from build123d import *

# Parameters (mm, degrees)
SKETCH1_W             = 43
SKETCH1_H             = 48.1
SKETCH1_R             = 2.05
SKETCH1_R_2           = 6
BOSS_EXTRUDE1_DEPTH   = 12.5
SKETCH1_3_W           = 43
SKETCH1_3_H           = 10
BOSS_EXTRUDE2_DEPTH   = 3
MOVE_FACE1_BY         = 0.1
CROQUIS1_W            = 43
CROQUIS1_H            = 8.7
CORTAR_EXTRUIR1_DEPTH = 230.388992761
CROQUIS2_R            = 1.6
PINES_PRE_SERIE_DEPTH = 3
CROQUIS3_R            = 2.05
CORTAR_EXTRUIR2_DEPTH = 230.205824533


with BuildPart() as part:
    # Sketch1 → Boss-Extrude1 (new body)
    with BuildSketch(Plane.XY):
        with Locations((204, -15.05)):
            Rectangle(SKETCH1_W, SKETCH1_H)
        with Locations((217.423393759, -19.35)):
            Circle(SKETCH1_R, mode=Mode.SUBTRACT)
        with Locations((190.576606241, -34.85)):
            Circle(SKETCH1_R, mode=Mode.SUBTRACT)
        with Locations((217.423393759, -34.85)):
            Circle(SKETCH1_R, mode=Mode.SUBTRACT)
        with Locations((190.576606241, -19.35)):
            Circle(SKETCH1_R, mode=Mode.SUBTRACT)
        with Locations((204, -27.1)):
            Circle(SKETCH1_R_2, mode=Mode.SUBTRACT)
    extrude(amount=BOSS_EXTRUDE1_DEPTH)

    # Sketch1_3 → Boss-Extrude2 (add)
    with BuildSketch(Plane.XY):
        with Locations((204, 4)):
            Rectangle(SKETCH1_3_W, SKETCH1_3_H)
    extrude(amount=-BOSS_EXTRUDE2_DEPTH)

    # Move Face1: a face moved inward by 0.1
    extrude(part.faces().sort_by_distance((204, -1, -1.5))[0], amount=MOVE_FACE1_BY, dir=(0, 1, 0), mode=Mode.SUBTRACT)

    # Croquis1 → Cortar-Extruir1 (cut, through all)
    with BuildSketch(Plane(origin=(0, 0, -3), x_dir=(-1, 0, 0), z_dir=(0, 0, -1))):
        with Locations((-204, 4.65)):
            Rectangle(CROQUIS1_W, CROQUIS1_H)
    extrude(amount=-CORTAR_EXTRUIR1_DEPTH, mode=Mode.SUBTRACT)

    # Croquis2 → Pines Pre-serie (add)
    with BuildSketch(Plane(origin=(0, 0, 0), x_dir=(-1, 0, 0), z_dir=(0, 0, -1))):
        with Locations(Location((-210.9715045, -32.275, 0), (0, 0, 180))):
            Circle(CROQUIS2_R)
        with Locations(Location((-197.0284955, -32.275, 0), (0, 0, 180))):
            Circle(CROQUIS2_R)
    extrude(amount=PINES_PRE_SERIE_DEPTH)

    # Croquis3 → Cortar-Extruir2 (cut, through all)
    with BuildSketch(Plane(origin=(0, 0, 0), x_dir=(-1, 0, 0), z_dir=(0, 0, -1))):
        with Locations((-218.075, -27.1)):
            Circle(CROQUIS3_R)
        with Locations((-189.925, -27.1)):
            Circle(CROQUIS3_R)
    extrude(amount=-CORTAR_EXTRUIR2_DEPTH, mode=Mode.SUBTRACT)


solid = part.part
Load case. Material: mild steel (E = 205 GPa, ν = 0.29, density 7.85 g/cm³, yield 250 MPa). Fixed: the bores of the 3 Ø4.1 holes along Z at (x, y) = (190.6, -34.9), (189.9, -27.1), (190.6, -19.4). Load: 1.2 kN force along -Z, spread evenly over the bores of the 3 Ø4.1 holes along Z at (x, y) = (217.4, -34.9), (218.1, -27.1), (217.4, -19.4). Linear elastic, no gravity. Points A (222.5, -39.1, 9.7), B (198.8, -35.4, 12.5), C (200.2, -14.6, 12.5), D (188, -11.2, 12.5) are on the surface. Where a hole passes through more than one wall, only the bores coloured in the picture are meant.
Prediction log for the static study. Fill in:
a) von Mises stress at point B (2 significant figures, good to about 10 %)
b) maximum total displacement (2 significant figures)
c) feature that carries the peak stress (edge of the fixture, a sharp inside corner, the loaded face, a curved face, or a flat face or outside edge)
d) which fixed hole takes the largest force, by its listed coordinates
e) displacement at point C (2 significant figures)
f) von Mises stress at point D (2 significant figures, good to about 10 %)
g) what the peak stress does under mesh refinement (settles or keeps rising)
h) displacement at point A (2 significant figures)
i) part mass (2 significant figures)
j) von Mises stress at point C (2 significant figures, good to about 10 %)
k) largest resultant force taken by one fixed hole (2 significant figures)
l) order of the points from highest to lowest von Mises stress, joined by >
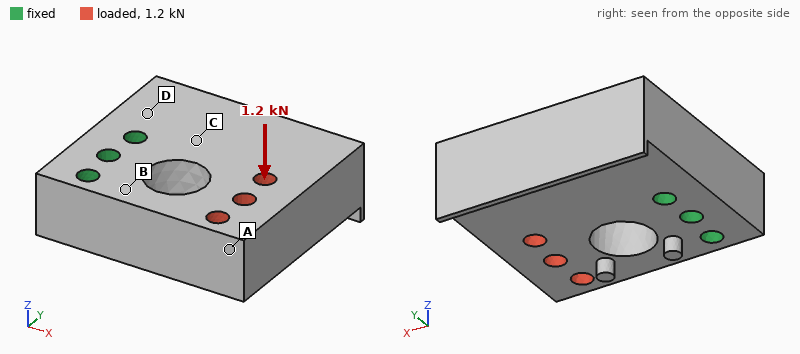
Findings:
47 MPa
17 µm
edge of the fixture
(190.6, -19.4)
2.9 µm
15 MPa
keeps rising
15 µm
150 g
25 MPa
500 N
B > C > D > A
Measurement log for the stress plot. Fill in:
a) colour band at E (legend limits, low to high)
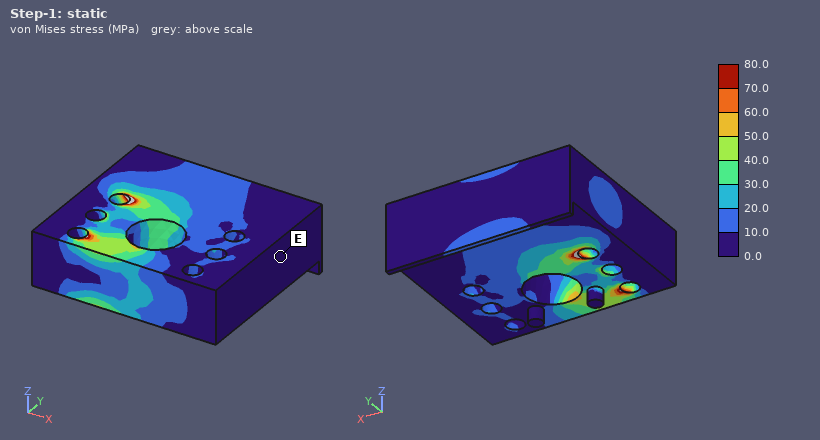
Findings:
0.0 to 10.0 MPa
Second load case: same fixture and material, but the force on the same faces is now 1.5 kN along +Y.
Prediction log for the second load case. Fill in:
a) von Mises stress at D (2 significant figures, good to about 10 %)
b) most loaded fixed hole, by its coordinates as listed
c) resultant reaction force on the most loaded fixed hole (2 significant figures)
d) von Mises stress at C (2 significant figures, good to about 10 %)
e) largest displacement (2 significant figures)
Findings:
9.6 MPa
(190.6, -19.4)
2.3 kN
14 MPa
8.7 µm
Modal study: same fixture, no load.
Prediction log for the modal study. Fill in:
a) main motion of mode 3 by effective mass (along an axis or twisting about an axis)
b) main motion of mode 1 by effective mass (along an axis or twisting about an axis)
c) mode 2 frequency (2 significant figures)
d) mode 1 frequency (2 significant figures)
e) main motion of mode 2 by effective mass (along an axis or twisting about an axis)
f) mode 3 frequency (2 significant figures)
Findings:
twisting about X
along Z
8500 Hz
6300 Hz
along Y
11 kHz
